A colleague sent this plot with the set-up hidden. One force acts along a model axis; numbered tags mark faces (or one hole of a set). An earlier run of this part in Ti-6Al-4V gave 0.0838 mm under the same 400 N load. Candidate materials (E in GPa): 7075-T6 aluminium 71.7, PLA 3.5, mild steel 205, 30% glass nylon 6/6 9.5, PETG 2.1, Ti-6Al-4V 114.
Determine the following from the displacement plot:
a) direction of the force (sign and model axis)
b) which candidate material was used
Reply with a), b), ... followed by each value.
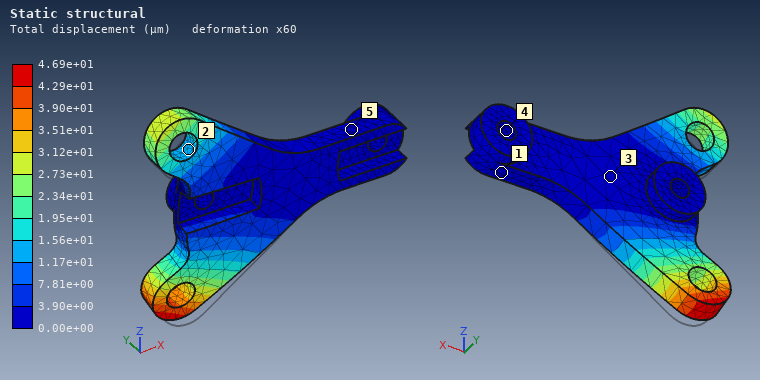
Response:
a) +Y
b) mild steel
